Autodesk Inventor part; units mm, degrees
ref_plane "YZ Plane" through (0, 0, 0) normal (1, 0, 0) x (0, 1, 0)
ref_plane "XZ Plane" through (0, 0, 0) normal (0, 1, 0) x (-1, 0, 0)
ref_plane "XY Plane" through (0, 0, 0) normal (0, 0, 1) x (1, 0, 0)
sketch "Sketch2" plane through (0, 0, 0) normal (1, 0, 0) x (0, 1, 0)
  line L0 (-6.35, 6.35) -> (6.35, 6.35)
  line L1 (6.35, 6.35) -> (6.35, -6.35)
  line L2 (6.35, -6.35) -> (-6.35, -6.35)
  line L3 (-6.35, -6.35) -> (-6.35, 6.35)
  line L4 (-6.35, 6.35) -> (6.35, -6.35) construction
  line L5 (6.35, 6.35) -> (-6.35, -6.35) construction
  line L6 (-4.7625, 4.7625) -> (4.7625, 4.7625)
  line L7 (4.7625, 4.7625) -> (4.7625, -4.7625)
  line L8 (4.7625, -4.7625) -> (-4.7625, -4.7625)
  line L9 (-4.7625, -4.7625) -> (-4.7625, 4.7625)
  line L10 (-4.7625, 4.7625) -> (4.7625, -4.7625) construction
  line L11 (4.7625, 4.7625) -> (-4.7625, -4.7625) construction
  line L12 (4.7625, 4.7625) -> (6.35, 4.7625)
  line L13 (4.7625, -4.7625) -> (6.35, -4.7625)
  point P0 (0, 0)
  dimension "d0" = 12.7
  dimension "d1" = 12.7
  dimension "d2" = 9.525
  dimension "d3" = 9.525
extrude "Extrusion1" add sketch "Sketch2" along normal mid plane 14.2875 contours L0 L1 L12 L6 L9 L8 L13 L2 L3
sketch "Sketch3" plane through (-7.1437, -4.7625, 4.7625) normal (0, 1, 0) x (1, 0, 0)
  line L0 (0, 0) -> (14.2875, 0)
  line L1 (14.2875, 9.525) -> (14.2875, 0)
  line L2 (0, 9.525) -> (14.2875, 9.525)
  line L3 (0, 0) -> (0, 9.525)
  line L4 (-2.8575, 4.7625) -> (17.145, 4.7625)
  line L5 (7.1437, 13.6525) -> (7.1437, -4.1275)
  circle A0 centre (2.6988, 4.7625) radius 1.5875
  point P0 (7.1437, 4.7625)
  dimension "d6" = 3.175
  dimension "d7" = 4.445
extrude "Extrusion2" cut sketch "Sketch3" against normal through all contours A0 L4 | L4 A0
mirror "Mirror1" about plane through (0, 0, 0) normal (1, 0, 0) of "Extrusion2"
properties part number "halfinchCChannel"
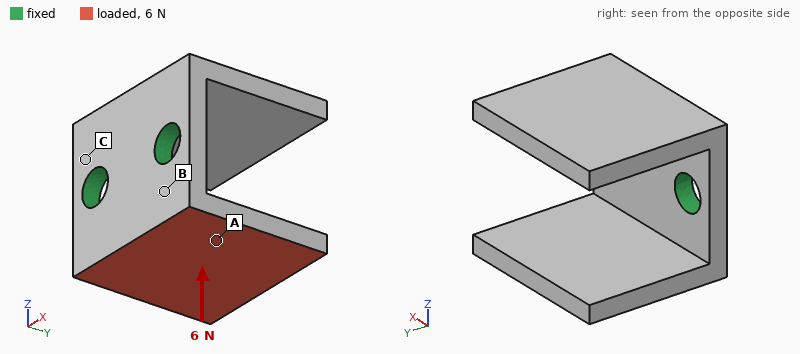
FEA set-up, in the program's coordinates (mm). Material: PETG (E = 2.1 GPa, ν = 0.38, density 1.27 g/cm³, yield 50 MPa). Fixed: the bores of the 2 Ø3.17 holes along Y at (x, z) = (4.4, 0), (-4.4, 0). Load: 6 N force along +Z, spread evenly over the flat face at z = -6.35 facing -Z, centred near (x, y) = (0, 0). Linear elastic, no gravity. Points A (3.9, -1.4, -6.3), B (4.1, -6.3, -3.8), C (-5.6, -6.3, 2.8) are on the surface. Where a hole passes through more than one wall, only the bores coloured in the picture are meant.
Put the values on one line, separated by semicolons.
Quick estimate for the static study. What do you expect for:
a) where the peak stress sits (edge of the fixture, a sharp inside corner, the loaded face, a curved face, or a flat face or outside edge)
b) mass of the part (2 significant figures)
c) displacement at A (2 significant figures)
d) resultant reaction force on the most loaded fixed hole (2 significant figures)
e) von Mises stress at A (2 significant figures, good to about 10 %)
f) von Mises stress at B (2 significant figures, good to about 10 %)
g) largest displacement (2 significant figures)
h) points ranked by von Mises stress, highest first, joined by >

a flat face or outside edge; 0.97 g; 0.085 mm; 3.2 N; 2.2 MPa; 4.7 MPa; 0.26 mm; B > A > C
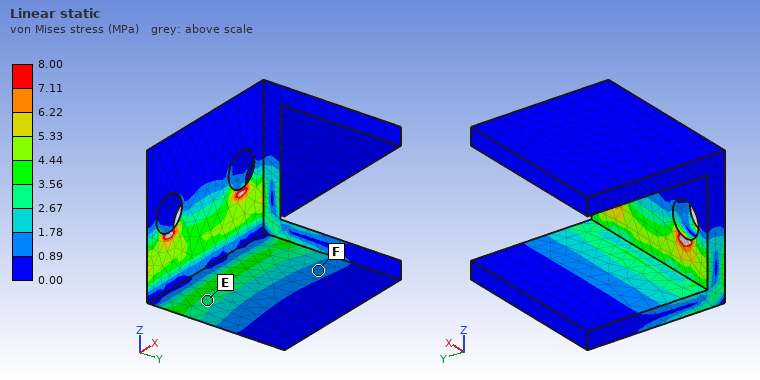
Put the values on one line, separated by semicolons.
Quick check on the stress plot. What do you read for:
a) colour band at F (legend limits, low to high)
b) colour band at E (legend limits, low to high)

0.89 to 1.78 MPa; 2.67 to 3.56 MPa
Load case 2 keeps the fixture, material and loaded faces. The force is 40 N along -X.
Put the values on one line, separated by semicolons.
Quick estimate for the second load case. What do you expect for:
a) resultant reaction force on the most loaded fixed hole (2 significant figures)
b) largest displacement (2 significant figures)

36 N; 0.24 mm
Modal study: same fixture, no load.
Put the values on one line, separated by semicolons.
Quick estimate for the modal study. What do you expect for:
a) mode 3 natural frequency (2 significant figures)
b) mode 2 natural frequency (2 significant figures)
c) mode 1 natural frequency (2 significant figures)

3300 Hz; 1500 Hz; 1500 Hz
